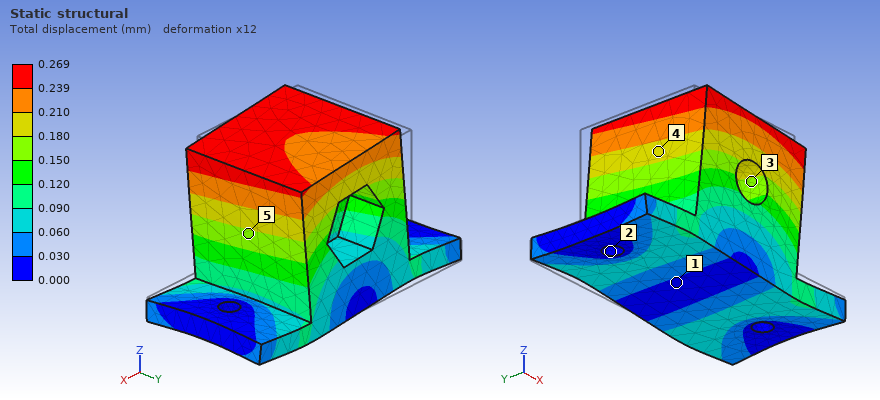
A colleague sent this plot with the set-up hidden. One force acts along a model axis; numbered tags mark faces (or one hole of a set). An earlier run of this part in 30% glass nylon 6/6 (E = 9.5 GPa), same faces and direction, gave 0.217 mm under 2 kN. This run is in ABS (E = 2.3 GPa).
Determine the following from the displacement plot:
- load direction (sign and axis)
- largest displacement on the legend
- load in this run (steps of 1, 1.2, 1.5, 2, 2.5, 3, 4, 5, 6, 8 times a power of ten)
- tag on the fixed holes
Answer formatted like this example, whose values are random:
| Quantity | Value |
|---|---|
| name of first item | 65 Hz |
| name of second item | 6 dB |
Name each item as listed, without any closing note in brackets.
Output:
| Quantity | Value |
|---|---|
| load direction | +X |
| largest displacement on the legend | 0.269 mm |
| load in this run | 600 N |
| tag on the fixed holes | 2 |
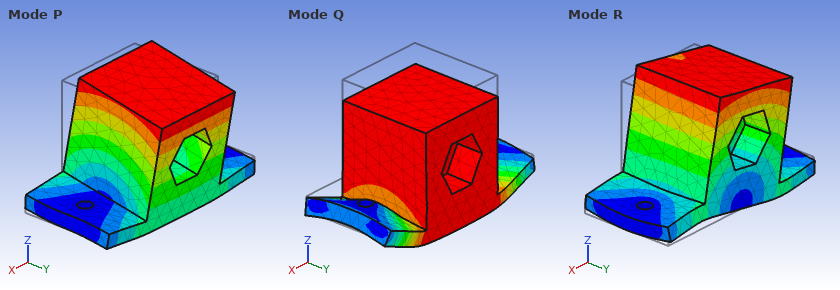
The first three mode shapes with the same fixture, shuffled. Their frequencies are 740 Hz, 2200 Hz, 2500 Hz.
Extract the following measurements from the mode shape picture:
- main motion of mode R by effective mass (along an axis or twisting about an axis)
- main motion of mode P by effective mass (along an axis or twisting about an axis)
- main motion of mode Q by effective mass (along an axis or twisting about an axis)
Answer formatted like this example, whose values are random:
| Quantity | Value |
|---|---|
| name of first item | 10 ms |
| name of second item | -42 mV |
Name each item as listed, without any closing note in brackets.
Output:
| Quantity | Value |
|---|---|
| main motion of mode R by effective mass | along X |
| main motion of mode P by effective mass | along Y |
| main motion of mode Q by effective mass | along Z |
